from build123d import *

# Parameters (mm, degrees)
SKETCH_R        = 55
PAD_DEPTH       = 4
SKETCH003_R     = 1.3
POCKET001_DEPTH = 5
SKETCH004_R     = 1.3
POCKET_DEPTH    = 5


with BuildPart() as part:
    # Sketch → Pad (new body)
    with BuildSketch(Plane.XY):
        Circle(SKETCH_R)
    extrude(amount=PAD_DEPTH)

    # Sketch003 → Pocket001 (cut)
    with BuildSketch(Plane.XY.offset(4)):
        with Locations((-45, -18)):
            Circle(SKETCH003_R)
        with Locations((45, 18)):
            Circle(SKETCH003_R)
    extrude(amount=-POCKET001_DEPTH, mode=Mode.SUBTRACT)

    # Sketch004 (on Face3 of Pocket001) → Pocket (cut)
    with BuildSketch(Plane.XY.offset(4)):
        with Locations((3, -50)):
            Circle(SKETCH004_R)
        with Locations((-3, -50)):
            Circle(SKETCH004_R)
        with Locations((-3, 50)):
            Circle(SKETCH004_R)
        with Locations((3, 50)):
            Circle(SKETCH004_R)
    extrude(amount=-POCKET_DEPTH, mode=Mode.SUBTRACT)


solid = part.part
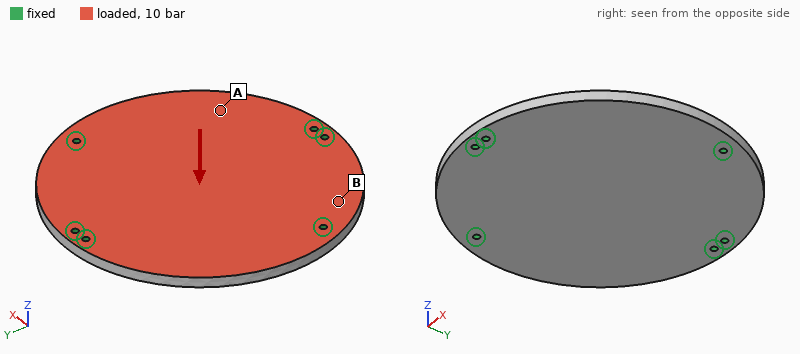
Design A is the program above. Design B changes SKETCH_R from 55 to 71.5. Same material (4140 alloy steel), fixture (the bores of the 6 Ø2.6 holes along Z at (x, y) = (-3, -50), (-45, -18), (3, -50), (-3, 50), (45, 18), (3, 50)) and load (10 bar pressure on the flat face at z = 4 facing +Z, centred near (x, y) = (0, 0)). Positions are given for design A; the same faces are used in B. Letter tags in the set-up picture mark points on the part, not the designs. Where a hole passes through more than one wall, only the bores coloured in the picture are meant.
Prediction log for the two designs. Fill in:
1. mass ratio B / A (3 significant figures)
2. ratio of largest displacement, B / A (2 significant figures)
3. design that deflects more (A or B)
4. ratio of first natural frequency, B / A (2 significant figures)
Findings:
1.69
2.4
B
0.68
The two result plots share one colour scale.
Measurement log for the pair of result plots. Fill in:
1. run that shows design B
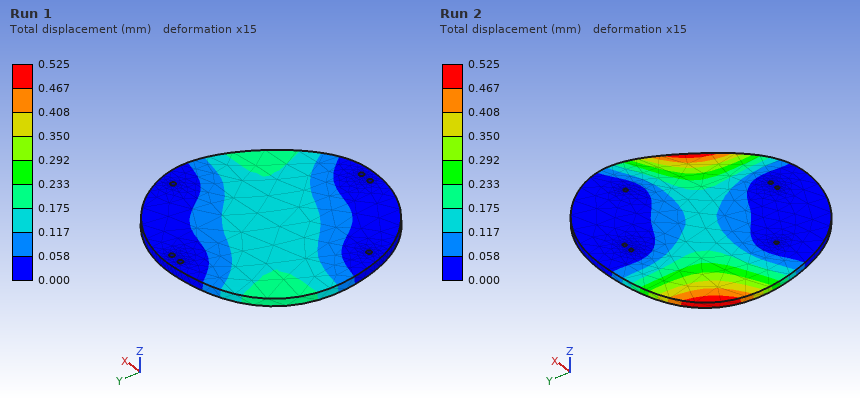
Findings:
Run 2
